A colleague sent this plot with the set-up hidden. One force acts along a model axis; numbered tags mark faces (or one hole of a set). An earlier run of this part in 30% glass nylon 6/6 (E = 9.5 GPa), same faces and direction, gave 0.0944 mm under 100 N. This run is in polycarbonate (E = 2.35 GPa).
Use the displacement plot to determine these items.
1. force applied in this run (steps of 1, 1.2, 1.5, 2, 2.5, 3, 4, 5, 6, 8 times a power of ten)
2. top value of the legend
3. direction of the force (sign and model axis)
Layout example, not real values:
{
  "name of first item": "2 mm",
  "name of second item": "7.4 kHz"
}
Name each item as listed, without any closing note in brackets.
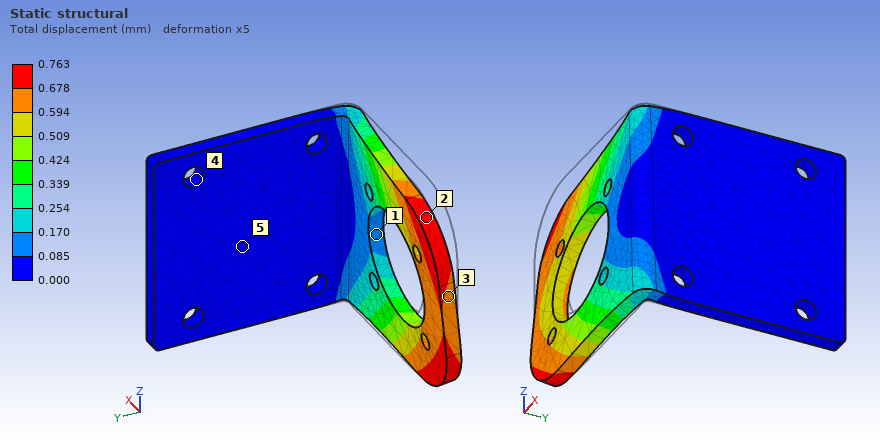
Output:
{
  "force applied in this run": "200 N",
  "top value of the legend": "0.763 mm",
  "direction of the force": "-Z"
}
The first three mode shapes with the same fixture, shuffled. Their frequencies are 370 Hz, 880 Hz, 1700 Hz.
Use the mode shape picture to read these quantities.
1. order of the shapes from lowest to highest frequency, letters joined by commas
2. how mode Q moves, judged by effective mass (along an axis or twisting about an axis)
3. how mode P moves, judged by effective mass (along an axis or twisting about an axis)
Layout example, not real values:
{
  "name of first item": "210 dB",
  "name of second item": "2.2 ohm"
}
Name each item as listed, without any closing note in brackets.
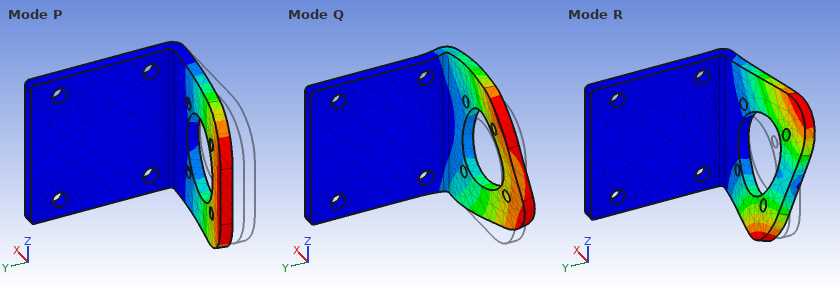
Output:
{
  "order of the shapes from lowest to highest frequency, letters joined by commas": "P, R, Q",
  "how mode Q moves, judged by effective mass": "along Z",
  "how mode P moves, judged by effective mass": "along Y"
}
